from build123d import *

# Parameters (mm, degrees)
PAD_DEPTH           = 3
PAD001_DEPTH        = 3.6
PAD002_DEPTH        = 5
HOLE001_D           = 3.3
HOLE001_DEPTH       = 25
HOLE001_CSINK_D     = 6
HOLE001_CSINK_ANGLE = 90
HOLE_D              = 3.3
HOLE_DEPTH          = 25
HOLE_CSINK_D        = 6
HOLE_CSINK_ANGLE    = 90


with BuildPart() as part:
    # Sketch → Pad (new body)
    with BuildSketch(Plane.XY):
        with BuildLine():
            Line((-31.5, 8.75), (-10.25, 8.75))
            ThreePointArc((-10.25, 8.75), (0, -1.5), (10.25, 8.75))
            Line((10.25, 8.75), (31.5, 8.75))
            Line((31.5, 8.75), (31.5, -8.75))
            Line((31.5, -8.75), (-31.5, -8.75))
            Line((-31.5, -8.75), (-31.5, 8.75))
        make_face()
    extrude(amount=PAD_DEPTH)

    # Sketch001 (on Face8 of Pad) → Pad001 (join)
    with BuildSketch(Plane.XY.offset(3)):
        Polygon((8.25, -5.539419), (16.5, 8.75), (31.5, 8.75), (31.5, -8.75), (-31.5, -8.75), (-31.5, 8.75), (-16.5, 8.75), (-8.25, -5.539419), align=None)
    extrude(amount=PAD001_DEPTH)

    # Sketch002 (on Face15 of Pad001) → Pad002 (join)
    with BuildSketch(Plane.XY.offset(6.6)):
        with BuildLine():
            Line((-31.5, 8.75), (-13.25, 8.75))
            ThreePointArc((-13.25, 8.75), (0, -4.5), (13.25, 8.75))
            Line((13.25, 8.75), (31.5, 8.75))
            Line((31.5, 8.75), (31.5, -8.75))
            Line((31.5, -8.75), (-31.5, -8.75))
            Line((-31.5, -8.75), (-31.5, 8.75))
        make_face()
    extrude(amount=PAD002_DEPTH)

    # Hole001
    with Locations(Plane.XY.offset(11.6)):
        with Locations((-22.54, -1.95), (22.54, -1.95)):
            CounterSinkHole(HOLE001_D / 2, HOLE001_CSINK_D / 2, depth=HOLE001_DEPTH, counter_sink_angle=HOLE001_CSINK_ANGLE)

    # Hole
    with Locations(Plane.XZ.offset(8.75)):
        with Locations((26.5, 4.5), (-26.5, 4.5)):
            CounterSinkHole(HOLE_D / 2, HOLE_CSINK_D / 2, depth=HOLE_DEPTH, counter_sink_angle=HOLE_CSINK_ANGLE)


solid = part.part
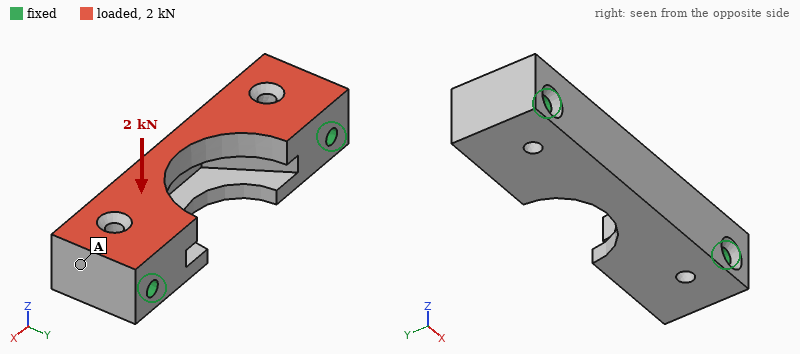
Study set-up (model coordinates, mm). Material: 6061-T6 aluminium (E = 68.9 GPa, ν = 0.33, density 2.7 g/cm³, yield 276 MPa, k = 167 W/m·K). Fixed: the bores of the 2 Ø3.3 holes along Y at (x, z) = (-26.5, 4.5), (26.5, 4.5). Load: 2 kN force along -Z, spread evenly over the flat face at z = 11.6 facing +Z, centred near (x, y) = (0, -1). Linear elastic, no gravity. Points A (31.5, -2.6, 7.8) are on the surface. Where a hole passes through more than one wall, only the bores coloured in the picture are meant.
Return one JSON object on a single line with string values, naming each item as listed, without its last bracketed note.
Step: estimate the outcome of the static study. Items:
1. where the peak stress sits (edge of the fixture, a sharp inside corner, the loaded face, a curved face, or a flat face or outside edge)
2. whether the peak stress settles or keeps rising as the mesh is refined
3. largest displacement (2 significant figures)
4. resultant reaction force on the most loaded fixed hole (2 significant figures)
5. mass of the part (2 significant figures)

{"where the peak stress sits": "edge of the fixture", "whether the peak stress settles or keeps rising as the mesh is refined": "keeps rising", "largest displacement": "13 µm", "resultant reaction force on the most loaded fixed hole": "1.0 kN", "mass of the part": "25 g"}
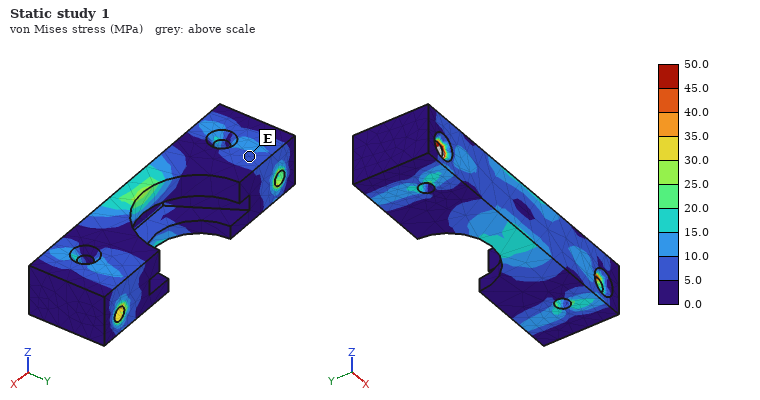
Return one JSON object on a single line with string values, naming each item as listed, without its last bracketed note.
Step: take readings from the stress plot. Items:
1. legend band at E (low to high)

{"legend band at E": "5.0 to 10.0 MPa"}
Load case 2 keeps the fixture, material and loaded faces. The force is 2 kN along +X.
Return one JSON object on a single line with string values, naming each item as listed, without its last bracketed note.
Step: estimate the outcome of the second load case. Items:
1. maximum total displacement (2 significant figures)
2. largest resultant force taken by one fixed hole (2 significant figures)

{"maximum total displacement": "4.4 µm", "largest resultant force taken by one fixed hole": "1.0 kN"}
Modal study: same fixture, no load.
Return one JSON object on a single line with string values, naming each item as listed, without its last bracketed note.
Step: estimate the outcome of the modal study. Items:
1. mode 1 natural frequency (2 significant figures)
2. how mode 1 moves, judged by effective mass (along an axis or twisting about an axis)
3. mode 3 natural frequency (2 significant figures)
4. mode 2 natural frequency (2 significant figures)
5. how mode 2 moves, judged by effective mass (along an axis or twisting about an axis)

{"mode 1 natural frequency": "15 kHz", "how mode 1 moves, judged by effective mass": "along Z", "mode 3 natural frequency": "27 kHz", "mode 2 natural frequency": "24 kHz", "how mode 2 moves, judged by effective mass": "along Y"}
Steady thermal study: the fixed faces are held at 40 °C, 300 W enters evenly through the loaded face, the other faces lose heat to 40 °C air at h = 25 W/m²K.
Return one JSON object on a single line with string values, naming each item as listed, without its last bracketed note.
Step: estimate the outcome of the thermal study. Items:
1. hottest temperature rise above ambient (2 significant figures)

{"hottest temperature rise above ambient": "63 K"}
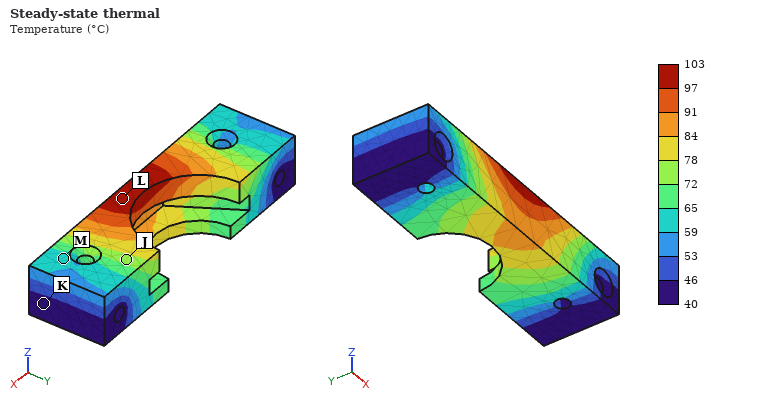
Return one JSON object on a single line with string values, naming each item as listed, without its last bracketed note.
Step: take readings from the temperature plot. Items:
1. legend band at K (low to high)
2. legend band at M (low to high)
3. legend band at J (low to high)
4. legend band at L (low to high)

{"legend band at K": "40 to 46 °C", "legend band at M": "59 to 65 °C", "legend band at J": "72 to 78 °C", "legend band at L": "97 to 103 °C"}
